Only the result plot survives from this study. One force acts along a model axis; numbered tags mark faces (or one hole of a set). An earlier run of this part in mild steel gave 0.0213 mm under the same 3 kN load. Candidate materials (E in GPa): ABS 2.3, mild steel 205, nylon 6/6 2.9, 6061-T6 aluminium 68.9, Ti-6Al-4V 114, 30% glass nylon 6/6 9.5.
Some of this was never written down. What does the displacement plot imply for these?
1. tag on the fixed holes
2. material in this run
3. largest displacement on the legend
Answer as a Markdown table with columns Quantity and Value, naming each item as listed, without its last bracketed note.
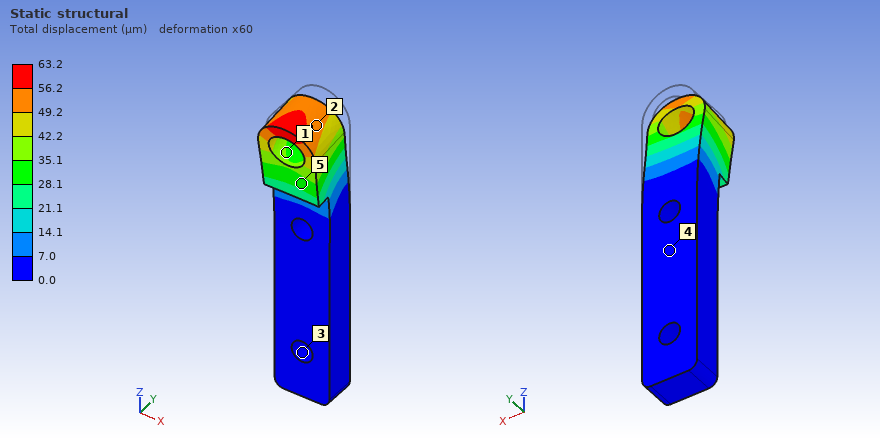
| Quantity | Value |
|---|---|
| tag on the fixed holes | 3 |
| material in this run | 6061-T6 aluminium |
| largest displacement on the legend | 63.2 µm |
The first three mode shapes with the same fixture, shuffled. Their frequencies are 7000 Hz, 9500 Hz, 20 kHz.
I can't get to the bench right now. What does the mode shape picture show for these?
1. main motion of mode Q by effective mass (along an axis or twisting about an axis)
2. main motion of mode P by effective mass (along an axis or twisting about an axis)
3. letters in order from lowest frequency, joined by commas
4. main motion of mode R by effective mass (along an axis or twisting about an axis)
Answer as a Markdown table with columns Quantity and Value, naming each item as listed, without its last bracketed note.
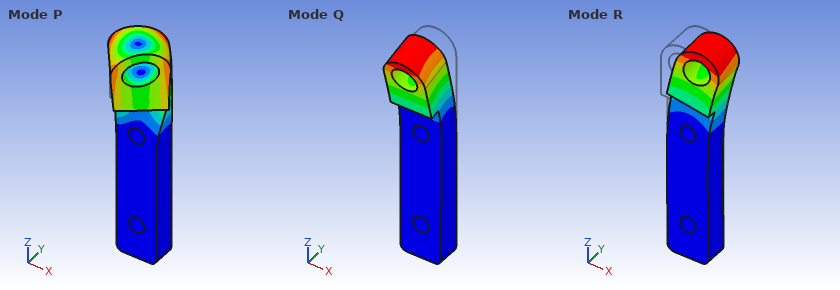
| Quantity | Value |
|---|---|
| main motion of mode Q by effective mass | along Y |
| main motion of mode P by effective mass | twisting about Z |
| letters in order from lowest frequency, joined by commas | Q, R, P |
| main motion of mode R by effective mass | along X |
